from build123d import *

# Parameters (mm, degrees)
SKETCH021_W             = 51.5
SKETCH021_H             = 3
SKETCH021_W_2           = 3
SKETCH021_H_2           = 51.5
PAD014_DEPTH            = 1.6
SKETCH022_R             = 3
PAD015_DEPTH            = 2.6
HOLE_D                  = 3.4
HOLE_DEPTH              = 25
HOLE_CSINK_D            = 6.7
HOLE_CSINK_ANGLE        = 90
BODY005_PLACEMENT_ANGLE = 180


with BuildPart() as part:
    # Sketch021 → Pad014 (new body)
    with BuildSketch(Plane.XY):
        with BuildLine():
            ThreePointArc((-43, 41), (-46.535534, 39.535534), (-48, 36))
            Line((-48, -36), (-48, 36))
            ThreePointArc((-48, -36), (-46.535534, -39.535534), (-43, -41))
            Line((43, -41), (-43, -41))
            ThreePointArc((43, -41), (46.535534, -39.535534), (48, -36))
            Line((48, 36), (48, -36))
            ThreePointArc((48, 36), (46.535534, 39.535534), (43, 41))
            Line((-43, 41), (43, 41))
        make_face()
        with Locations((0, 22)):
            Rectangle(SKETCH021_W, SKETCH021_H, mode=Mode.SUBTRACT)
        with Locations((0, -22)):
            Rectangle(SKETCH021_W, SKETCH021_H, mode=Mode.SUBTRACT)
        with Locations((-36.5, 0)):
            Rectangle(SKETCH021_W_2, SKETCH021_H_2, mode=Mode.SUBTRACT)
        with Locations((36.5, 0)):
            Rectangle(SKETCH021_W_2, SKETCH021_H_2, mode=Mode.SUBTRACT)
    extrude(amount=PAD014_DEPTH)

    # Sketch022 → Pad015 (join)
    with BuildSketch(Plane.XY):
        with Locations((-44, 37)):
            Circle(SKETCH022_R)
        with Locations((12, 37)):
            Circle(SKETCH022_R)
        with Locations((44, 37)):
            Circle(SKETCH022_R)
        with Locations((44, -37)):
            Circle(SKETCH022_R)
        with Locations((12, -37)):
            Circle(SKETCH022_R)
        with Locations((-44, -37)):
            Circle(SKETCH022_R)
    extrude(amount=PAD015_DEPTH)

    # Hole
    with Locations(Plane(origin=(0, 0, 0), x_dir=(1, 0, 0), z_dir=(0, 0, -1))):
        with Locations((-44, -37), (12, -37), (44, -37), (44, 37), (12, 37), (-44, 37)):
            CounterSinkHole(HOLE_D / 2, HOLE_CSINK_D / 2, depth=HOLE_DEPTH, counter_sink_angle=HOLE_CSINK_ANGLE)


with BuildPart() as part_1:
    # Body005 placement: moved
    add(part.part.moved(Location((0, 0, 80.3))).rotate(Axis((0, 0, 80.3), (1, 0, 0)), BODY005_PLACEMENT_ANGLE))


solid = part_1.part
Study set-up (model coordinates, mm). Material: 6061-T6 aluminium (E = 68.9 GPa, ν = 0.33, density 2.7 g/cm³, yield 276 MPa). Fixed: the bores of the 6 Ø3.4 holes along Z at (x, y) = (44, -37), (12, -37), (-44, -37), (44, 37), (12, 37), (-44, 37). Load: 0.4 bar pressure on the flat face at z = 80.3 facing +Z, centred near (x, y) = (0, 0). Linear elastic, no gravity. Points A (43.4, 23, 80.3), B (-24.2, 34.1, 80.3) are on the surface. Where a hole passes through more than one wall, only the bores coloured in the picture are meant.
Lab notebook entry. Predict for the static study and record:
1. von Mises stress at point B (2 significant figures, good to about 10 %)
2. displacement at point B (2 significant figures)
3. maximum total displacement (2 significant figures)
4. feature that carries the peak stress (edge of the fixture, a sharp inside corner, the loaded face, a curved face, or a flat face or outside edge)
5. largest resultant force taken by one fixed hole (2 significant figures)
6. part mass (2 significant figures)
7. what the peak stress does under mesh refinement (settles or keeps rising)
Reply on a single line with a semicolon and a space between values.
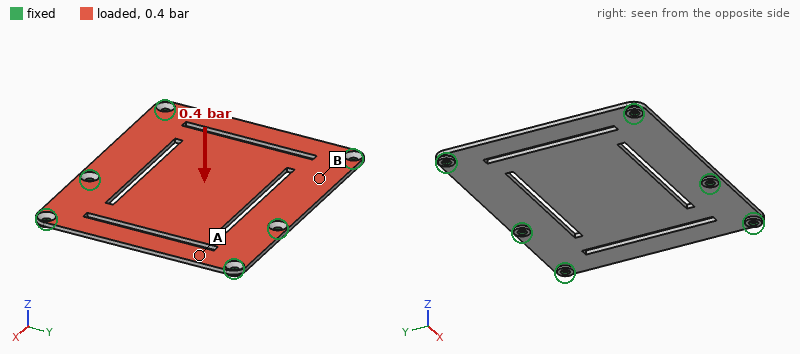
26 MPa; 0.086 mm; 0.37 mm; edge of the fixture; 130 N; 31 g; keeps rising
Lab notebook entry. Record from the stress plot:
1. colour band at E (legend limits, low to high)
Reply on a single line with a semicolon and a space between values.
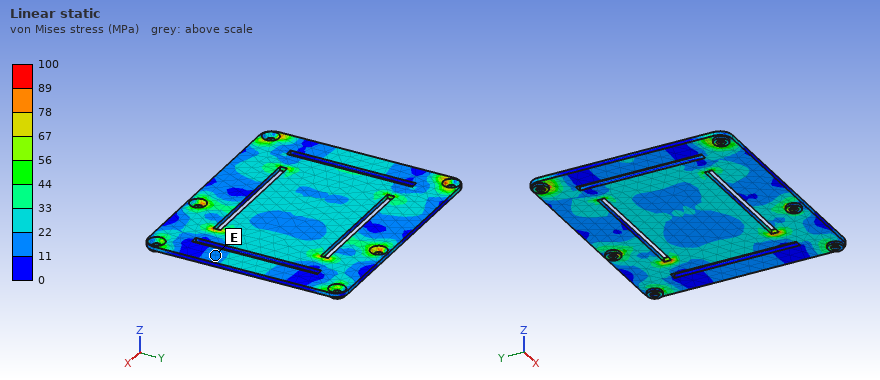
11 to 22 MPa
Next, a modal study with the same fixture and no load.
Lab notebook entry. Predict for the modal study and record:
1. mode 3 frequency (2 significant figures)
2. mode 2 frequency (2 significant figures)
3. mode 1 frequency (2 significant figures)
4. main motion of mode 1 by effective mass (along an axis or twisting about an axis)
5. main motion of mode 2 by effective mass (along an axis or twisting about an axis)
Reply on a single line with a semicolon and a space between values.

1800 Hz; 1500 Hz; 940 Hz; along Z; twisting about Y
